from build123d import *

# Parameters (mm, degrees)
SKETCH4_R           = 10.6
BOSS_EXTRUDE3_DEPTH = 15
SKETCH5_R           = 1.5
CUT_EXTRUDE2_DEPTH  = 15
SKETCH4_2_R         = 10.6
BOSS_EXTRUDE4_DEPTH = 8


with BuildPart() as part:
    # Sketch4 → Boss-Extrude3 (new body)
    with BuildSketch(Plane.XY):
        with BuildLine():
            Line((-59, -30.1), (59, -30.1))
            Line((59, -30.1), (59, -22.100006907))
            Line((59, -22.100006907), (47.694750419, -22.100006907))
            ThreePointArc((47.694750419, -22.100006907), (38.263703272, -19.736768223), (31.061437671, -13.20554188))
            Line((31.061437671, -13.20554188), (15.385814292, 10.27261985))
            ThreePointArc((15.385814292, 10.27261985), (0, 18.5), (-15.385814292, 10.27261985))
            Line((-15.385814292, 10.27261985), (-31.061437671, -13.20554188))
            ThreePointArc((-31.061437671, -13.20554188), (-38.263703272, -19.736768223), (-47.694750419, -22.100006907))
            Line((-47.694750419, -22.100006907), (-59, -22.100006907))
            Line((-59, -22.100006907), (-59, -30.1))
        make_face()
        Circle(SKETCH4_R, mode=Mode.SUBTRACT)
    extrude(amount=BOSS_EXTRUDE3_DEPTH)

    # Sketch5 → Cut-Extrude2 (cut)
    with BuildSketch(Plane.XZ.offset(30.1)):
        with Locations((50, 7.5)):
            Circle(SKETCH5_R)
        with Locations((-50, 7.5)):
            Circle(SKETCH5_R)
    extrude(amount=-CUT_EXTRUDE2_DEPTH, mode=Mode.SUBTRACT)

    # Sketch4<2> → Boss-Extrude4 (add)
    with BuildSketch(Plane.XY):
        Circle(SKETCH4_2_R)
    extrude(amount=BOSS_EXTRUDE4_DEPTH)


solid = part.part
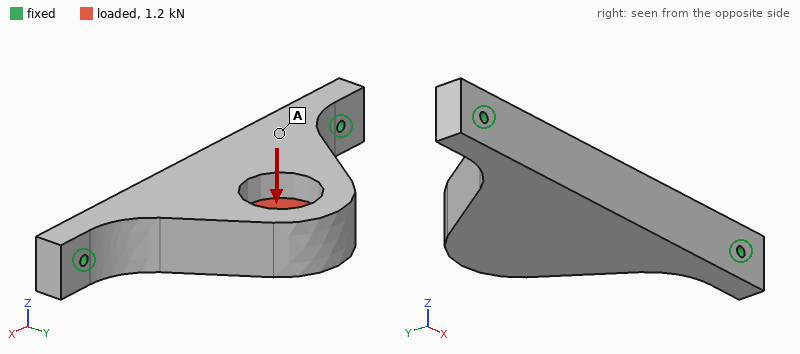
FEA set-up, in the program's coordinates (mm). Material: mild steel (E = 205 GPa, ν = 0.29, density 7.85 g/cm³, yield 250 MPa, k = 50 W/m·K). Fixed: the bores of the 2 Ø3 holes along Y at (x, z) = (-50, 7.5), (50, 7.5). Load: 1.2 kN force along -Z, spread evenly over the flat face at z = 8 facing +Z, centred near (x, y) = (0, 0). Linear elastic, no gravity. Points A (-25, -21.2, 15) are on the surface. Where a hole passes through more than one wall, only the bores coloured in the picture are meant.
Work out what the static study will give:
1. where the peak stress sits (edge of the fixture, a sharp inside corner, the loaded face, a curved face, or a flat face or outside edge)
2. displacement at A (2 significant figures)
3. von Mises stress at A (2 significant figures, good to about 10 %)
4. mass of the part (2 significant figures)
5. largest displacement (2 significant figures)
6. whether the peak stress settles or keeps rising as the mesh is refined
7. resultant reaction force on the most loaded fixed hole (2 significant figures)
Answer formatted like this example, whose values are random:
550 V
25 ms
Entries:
edge of the fixture
21 µm
20 MPa
320 g
92 µm
keeps rising
600 N
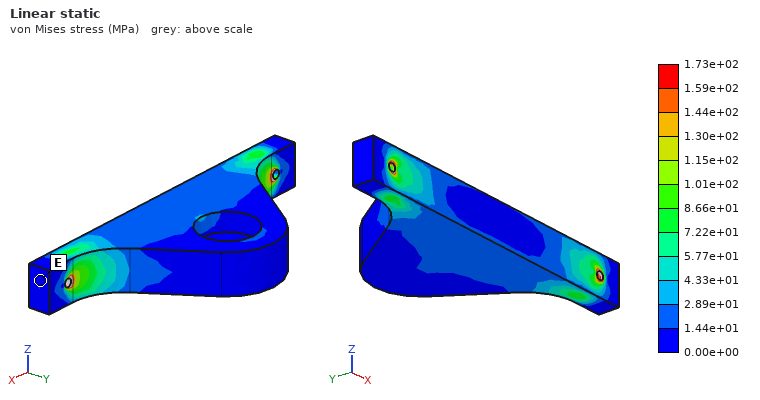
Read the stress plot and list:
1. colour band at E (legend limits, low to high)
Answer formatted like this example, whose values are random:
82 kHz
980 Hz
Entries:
0.00e+00 to 1.44e+01 MPa
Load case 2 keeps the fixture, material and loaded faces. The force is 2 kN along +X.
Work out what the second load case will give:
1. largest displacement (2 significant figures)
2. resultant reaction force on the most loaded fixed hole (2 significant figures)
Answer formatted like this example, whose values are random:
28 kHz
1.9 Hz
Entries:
4.6 µm
1.2 kN
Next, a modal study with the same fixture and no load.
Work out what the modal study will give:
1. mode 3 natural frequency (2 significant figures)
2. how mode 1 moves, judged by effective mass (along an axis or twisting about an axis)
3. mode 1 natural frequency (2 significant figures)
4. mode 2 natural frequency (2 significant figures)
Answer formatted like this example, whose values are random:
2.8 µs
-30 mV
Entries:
5400 Hz
along Z
1900 Hz
5300 Hz
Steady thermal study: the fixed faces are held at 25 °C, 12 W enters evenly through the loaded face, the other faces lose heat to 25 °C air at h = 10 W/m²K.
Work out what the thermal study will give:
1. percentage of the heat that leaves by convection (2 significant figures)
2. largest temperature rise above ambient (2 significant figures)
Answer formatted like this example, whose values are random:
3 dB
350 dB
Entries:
14 %
30 K
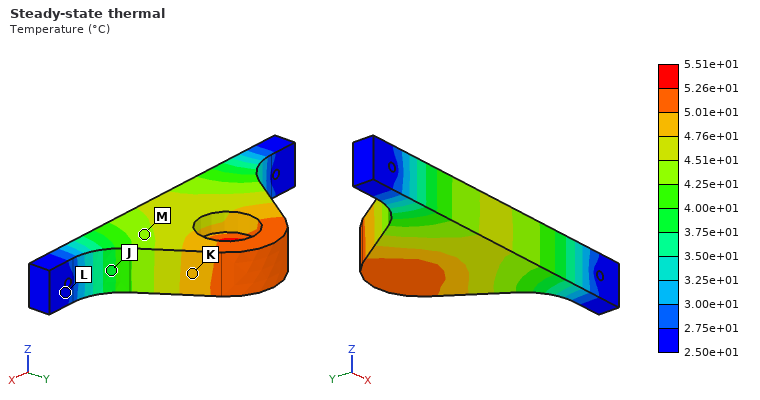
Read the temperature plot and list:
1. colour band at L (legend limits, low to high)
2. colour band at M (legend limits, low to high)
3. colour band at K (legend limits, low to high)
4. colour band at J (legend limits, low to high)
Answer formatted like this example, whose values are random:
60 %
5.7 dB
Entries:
2.50e+01 to 2.75e+01 °C
4.25e+01 to 4.51e+01 °C
4.76e+01 to 5.01e+01 °C
3.75e+01 to 4.00e+01 °C
